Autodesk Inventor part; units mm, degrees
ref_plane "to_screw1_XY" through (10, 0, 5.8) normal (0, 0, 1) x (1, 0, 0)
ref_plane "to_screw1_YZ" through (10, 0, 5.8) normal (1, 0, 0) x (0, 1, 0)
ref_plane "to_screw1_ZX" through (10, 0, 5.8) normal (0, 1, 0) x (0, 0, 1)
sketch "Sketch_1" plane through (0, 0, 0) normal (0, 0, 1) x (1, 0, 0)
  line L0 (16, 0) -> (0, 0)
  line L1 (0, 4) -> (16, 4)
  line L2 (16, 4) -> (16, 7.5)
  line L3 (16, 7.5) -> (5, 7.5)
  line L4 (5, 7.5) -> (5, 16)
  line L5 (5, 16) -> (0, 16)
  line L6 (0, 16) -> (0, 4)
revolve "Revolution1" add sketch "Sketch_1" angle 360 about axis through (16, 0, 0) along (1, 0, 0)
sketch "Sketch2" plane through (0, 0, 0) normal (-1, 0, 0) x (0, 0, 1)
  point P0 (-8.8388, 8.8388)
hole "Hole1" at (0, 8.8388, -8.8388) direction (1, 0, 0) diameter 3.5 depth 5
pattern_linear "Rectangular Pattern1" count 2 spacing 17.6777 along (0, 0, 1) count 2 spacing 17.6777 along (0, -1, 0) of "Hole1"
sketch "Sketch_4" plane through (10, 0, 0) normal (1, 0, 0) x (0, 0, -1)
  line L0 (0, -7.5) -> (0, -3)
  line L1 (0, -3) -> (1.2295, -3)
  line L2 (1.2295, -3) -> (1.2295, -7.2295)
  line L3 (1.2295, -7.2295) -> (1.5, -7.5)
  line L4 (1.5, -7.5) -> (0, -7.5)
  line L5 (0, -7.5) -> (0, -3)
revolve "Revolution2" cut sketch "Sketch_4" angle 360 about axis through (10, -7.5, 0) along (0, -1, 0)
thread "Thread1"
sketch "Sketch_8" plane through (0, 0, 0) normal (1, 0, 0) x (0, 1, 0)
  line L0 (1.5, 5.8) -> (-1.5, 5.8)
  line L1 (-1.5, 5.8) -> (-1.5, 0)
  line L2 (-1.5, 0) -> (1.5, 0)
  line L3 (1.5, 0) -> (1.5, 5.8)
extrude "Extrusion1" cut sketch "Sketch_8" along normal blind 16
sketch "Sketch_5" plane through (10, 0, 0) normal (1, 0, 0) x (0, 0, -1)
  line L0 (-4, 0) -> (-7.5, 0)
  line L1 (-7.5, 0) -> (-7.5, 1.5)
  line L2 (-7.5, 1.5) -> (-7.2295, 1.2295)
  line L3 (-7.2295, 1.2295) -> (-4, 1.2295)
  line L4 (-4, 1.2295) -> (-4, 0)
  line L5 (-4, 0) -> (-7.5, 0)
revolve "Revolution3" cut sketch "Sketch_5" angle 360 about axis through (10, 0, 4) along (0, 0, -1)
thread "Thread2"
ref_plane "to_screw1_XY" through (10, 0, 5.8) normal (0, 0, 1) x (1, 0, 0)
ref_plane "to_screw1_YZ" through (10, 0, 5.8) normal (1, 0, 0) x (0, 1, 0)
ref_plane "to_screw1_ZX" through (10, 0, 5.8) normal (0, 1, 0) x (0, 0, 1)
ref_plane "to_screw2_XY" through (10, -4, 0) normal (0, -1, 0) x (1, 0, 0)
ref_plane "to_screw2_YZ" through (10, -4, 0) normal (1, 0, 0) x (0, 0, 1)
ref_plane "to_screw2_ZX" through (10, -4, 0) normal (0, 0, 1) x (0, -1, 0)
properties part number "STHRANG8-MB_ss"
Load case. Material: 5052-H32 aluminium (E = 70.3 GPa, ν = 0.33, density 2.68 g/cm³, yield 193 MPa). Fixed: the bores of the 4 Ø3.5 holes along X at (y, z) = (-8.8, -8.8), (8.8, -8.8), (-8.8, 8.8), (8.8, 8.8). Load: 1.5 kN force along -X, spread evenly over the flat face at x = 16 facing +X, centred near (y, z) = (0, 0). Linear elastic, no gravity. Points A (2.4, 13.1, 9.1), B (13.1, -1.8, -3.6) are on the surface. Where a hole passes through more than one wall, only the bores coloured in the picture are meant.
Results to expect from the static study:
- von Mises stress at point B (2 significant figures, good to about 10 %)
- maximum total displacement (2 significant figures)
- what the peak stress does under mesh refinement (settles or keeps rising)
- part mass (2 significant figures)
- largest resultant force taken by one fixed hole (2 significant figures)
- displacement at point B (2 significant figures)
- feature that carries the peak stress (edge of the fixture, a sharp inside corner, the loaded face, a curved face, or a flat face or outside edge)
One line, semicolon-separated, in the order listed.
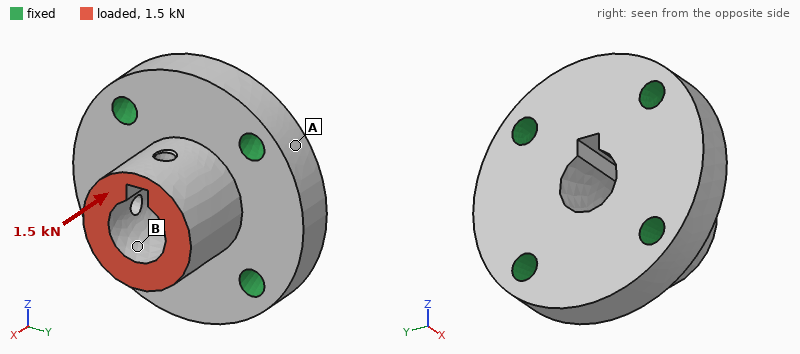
13 MPa; 5.4 µm; keeps rising; 13 g; 400 N; 4.4 µm; edge of the fixture
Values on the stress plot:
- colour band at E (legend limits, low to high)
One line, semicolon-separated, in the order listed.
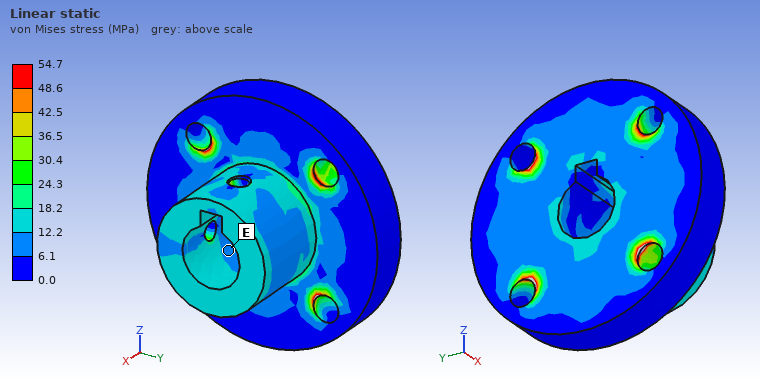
6.1 to 12.2 MPa
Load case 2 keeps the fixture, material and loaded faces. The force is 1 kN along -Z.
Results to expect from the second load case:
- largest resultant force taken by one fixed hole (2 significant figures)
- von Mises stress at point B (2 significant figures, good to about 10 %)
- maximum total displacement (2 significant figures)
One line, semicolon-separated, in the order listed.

500 N; 20 MPa; 20 µm
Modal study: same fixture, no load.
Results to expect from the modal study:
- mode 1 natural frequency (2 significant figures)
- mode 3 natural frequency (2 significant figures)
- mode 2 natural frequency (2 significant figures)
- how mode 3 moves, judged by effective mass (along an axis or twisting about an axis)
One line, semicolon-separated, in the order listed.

31 kHz; 43 kHz; 32 kHz; along X
